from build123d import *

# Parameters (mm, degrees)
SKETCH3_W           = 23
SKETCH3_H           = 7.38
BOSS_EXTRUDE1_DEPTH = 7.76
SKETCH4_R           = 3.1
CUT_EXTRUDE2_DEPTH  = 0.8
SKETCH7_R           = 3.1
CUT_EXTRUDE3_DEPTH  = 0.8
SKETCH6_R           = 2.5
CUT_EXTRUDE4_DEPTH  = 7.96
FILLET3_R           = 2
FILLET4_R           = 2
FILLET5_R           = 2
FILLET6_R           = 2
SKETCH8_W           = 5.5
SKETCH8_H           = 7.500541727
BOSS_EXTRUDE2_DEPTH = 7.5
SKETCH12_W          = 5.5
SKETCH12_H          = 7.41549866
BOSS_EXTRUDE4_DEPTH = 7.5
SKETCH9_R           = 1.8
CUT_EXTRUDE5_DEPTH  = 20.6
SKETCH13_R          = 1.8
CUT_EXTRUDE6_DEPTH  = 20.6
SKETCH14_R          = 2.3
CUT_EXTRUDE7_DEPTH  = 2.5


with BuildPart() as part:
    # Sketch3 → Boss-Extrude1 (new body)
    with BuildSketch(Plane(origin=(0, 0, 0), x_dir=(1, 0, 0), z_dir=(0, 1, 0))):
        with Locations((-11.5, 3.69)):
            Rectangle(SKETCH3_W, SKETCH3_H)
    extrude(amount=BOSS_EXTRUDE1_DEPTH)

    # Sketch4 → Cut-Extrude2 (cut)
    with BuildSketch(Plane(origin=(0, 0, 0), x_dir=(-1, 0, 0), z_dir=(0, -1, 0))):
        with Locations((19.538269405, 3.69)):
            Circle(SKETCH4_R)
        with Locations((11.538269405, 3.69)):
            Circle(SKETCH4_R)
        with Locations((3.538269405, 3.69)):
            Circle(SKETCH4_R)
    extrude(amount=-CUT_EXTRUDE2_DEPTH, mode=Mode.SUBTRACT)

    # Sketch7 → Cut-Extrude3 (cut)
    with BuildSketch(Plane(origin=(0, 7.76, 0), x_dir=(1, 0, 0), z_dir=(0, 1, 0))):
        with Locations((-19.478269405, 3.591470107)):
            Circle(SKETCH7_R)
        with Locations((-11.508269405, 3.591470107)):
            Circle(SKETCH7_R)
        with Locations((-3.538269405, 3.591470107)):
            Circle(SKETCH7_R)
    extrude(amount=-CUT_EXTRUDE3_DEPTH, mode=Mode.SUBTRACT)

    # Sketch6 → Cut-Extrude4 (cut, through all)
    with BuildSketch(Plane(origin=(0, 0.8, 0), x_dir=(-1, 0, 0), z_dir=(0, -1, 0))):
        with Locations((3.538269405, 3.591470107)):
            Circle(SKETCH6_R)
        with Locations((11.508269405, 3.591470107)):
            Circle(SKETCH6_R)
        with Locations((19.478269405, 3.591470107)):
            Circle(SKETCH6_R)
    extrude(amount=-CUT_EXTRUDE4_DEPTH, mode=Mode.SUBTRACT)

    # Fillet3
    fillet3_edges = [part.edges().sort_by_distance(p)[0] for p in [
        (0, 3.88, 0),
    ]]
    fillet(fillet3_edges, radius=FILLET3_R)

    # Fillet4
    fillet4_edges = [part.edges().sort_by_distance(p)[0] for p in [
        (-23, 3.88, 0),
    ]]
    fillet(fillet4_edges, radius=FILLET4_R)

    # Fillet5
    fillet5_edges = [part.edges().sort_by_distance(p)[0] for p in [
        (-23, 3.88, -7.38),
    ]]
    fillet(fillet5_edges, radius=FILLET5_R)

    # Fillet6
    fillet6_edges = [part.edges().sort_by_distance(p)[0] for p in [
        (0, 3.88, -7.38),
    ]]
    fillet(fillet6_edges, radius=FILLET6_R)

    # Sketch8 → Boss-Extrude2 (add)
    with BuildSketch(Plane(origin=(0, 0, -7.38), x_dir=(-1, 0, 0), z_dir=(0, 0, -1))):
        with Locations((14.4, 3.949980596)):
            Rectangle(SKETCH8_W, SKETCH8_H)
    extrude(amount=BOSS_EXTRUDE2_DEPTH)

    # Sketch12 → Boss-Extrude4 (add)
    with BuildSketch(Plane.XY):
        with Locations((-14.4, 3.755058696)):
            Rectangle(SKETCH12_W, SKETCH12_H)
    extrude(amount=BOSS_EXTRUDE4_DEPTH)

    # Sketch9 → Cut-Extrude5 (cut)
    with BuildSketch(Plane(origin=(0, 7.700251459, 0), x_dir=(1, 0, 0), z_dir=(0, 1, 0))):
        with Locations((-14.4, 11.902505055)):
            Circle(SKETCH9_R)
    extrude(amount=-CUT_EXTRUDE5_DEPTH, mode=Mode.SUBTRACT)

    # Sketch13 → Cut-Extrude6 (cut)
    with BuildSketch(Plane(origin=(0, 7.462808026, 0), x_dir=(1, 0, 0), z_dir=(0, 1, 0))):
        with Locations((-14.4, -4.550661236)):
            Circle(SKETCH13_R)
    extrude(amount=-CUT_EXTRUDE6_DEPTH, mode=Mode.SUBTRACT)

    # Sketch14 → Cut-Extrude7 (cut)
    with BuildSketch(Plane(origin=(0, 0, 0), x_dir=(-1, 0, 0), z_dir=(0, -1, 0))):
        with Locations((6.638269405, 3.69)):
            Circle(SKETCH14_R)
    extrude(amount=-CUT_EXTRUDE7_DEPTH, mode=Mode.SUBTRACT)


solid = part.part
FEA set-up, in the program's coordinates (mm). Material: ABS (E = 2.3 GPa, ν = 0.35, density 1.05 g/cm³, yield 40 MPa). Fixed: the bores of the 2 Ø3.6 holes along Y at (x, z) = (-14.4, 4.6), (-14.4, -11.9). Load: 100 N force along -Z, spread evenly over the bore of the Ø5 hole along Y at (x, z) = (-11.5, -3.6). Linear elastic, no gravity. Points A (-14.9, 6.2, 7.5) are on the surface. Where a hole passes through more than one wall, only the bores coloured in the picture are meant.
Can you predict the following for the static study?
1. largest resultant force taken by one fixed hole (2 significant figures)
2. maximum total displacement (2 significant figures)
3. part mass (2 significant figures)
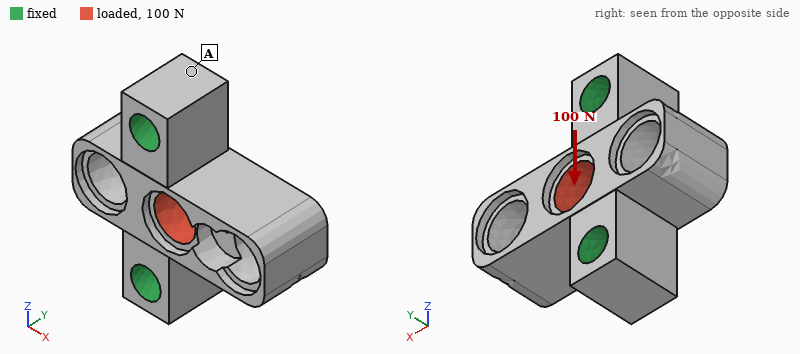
54 N
28 µm
1.3 g
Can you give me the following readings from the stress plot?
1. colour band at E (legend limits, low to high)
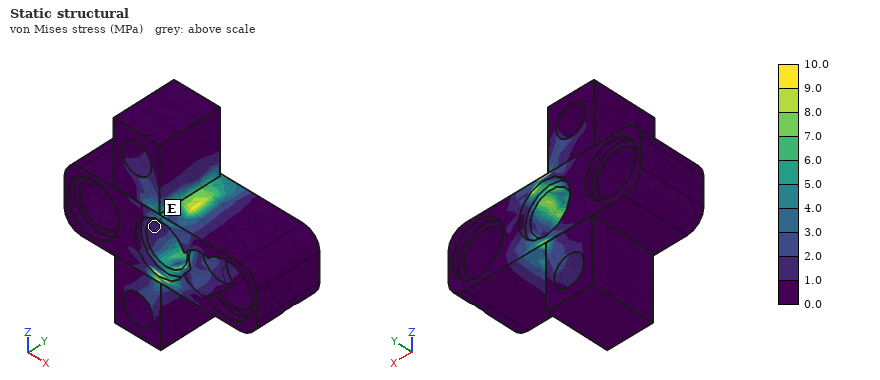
1.0 to 2.0 MPa
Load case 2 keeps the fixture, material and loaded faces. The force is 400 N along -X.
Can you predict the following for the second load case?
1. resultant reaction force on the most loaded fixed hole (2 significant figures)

200 N
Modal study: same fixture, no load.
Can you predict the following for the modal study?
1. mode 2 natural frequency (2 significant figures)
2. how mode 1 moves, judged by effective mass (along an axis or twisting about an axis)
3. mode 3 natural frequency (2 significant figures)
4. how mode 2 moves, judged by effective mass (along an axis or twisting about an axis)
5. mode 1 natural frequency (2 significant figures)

7100 Hz
along Y
10000 Hz
along Z
5700 Hz
